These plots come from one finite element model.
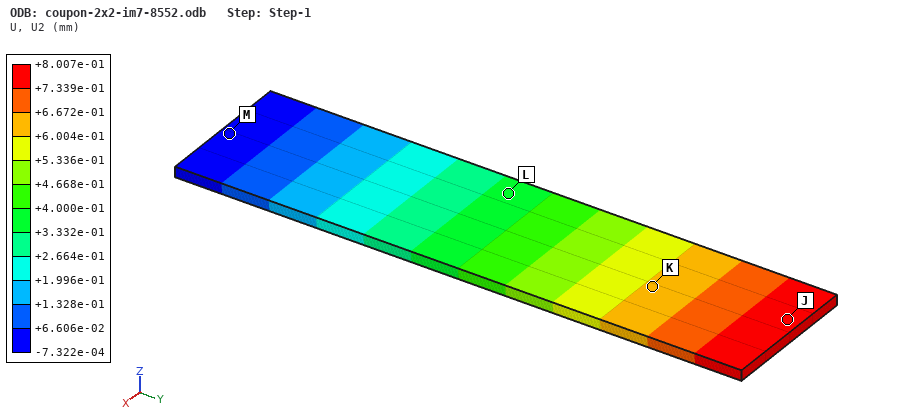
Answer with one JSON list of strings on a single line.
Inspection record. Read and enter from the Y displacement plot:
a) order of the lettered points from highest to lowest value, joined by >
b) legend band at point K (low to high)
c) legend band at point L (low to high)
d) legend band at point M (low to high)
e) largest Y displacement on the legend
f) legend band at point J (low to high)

["J > K > L > M", "+6.004e-01 to +6.672e-01 mm", "+3.332e-01 to +4.000e-01 mm", "-7.322e-04 to +6.606e-02 mm", "+8.007e-01 mm", "+7.339e-01 to +8.007e-01 mm"]
